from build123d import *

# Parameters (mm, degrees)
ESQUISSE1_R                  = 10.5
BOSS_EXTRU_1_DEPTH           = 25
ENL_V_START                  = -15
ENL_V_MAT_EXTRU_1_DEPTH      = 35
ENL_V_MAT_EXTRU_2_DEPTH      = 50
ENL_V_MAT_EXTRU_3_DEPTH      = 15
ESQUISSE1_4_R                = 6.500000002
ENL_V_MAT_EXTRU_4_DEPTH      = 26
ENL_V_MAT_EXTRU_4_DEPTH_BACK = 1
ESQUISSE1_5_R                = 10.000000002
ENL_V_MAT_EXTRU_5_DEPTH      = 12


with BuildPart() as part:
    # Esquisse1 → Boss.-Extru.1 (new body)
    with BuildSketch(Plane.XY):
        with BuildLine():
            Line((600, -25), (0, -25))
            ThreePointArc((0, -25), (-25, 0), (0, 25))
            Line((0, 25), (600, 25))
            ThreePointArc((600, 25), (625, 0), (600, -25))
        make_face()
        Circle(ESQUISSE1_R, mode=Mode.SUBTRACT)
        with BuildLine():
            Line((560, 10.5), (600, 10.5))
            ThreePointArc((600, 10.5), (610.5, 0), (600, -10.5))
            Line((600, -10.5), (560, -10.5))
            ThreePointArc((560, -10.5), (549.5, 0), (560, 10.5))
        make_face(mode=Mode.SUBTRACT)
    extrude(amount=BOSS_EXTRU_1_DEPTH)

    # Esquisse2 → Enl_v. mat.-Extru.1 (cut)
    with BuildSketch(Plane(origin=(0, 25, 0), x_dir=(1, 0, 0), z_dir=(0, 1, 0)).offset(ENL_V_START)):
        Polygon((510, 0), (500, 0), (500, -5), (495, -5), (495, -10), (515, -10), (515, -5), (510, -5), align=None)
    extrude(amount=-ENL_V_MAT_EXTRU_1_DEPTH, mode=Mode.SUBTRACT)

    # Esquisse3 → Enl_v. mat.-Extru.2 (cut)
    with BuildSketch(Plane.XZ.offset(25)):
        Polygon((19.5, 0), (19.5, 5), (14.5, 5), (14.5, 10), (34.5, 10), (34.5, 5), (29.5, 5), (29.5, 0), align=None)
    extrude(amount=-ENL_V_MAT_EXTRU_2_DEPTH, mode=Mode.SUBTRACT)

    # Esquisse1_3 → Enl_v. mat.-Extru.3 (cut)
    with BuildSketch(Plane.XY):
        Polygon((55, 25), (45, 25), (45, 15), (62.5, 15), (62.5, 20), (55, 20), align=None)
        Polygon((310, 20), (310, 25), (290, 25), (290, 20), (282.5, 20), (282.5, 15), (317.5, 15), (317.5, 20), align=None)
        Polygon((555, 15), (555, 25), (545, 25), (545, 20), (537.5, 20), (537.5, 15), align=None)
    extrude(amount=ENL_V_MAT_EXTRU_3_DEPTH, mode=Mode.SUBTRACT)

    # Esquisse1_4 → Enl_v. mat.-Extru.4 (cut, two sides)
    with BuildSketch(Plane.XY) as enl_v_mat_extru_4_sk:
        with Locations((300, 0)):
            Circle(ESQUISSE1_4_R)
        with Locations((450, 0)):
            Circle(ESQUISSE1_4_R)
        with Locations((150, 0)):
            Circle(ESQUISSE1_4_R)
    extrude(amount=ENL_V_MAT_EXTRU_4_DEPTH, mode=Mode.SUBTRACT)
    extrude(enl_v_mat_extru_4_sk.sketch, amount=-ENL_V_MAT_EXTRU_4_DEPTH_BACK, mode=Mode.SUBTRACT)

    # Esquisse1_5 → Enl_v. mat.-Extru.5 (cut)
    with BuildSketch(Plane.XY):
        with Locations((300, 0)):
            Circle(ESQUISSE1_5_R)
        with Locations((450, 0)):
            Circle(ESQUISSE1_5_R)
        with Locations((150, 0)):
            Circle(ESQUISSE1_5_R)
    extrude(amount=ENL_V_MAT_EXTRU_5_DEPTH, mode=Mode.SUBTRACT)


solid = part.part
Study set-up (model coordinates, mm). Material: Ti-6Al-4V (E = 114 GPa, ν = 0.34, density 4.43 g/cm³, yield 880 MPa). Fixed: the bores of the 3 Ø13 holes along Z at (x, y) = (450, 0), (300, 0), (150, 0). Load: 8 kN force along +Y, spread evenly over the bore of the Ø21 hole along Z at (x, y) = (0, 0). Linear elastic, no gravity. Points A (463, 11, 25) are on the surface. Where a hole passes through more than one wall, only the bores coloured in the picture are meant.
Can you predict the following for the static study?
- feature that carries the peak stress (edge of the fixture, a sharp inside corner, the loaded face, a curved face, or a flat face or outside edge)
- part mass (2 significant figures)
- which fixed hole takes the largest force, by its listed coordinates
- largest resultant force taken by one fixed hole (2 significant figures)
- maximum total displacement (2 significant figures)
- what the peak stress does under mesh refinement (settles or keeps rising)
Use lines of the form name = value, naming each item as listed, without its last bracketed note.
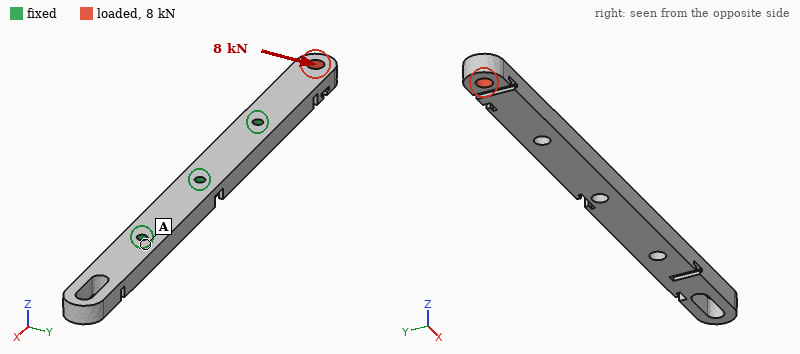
feature that carries the peak stress = edge of the fixture
part mass = 3.2 kg
which fixed hole takes the largest force, by its listed coordinates = (150, 0)
largest resultant force taken by one fixed hole = 14 kN
maximum total displacement = 0.68 mm
what the peak stress does under mesh refinement = keeps rising
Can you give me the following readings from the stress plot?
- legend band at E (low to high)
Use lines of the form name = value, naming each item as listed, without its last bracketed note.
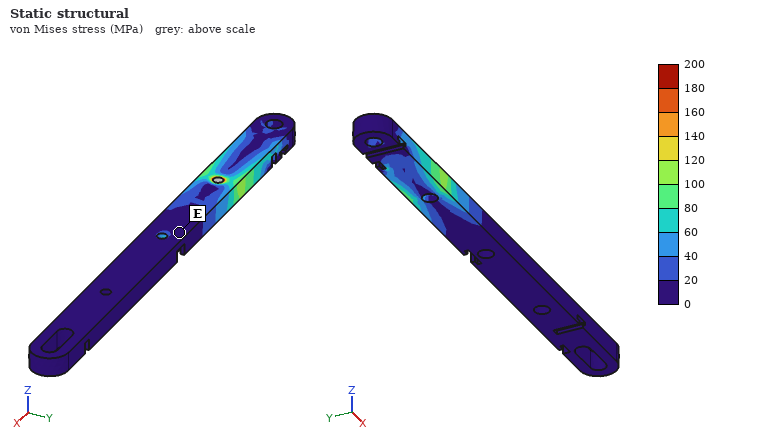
legend band at E = 0 to 20 MPa
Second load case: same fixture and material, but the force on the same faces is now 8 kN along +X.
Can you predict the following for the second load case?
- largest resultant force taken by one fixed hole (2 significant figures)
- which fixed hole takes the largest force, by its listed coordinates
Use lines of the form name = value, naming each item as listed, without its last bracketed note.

largest resultant force taken by one fixed hole = 6.8 kN
which fixed hole takes the largest force, by its listed coordinates = (150, 0)
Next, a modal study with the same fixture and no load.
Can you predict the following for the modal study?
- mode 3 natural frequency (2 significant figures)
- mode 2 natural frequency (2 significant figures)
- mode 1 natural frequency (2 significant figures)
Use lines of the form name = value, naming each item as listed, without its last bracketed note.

mode 3 natural frequency = 1100 Hz
mode 2 natural frequency = 640 Hz
mode 1 natural frequency = 630 Hz
